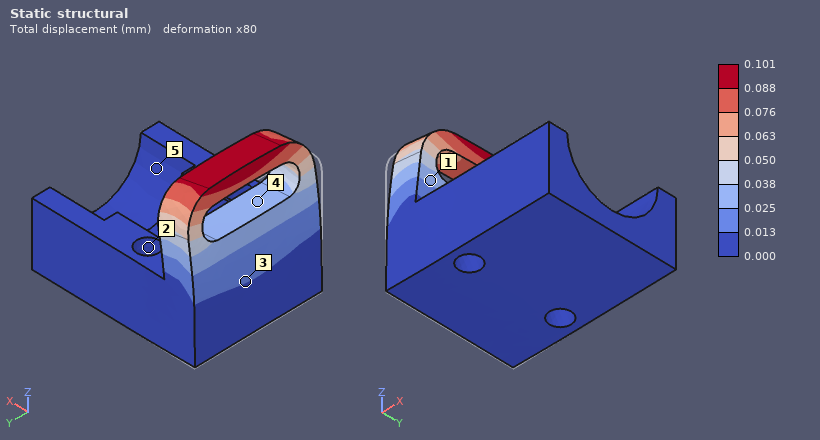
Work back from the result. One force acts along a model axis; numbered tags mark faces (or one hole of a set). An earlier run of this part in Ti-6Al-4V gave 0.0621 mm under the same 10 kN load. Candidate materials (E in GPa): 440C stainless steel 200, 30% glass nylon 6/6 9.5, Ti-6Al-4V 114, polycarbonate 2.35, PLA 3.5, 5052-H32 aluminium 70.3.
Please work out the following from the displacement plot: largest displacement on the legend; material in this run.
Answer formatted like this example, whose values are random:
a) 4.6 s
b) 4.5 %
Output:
a) 0.101 mm
b) 5052-H32 aluminium
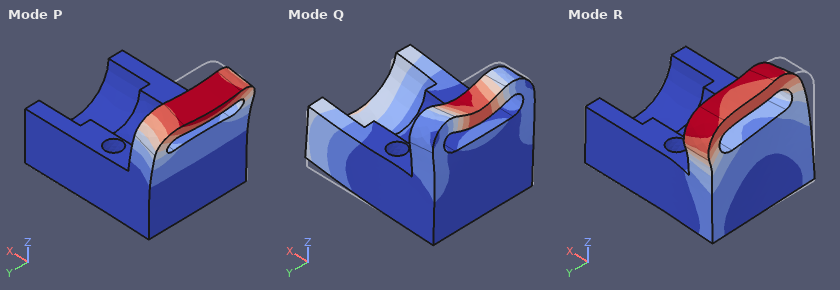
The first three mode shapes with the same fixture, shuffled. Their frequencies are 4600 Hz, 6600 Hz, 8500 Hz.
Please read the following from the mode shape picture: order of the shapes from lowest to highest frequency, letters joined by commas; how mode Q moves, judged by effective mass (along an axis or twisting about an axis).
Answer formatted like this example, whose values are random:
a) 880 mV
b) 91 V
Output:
a) P, R, Q
b) twisting about Y
